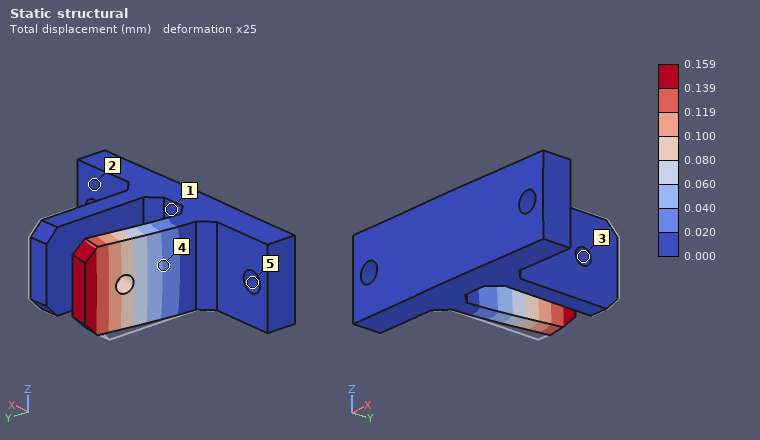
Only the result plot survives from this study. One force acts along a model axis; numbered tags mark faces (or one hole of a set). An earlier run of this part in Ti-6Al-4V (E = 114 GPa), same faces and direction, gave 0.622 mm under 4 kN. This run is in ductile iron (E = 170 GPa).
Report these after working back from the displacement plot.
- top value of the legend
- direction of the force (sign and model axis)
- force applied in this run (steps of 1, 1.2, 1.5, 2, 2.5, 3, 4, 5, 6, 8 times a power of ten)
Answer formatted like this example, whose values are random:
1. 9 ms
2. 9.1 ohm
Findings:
1. 0.159 mm
2. +X
3. 1.5 kN
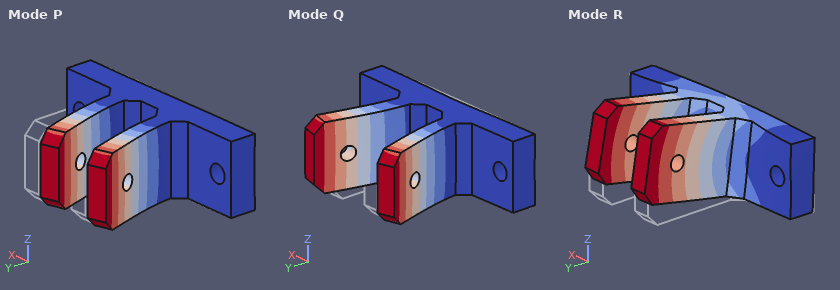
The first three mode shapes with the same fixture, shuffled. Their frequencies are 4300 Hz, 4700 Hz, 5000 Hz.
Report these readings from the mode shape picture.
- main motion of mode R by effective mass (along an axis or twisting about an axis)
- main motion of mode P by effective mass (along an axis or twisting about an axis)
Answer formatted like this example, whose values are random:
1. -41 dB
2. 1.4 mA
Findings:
1. along Z
2. along X
